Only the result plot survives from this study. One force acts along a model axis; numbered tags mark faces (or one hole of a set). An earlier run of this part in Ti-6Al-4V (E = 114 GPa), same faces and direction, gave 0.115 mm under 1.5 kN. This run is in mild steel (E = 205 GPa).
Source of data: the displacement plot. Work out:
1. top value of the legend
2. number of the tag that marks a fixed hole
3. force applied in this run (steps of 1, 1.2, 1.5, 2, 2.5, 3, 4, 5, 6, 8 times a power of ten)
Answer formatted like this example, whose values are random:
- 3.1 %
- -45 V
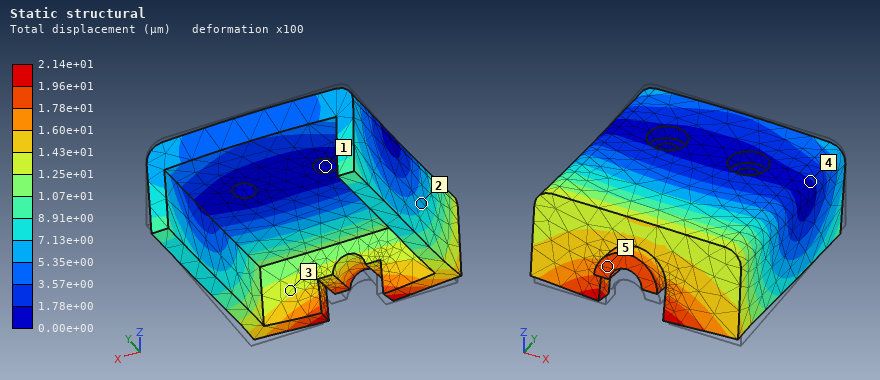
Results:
- 2.14e+01 µm
- 1
- 500 N
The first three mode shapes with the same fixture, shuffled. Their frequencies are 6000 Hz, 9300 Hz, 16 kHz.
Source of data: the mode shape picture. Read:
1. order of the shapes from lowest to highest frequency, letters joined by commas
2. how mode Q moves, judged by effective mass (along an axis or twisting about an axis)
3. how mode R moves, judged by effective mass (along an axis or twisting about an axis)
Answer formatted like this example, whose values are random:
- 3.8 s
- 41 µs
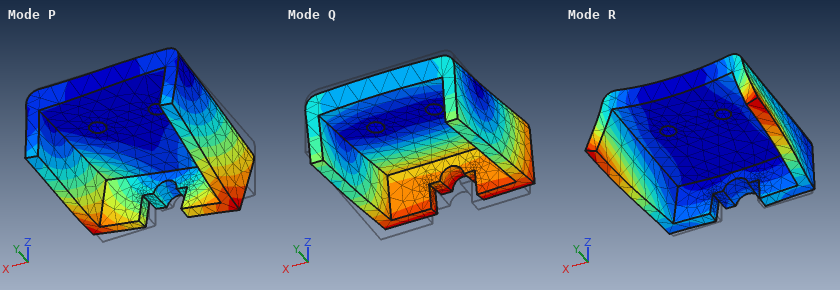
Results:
- Q, P, R
- along Z
- along Z
